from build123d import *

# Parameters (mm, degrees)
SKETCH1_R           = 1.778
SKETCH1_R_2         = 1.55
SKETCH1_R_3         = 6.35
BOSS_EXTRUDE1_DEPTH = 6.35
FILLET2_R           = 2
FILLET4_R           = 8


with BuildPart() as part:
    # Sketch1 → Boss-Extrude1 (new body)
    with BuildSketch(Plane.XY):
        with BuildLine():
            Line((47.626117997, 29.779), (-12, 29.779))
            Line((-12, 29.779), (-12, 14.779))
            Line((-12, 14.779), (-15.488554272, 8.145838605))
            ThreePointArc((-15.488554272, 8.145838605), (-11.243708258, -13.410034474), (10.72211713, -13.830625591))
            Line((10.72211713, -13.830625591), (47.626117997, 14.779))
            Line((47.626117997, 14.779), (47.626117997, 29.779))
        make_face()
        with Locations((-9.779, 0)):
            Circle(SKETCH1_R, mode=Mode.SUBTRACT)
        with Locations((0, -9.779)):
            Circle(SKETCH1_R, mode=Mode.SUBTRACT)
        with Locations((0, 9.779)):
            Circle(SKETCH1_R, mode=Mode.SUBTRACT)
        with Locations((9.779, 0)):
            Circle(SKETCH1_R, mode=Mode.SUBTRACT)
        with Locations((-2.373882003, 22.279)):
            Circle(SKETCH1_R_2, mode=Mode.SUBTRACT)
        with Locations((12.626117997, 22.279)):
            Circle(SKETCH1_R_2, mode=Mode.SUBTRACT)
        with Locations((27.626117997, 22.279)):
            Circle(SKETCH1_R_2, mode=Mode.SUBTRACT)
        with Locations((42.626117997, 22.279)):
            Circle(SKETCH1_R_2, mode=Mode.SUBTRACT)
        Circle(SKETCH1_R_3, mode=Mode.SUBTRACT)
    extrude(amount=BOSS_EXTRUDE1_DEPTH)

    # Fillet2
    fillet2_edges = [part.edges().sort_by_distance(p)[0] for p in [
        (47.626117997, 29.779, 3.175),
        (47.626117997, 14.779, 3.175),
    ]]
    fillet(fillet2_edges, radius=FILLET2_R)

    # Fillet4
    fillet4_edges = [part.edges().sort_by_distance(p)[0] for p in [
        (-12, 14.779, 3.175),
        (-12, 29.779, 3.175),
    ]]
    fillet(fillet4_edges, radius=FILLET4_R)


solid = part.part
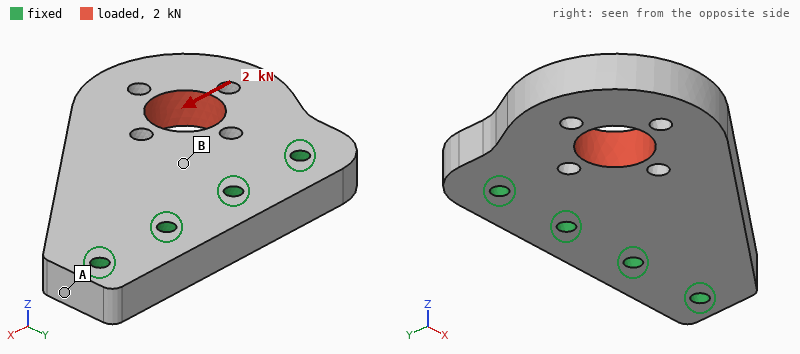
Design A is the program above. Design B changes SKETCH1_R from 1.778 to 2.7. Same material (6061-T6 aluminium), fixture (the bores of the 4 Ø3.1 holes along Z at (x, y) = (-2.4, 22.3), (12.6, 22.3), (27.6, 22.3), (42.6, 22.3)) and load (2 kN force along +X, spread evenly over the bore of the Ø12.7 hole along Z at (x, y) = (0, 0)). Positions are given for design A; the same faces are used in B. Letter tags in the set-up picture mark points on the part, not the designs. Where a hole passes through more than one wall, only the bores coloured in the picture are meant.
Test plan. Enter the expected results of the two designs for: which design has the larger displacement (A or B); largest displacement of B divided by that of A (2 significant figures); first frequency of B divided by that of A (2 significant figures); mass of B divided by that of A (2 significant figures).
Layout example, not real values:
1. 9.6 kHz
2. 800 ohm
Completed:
1. B
2. 1.2
3. 1.00
4. 0.97
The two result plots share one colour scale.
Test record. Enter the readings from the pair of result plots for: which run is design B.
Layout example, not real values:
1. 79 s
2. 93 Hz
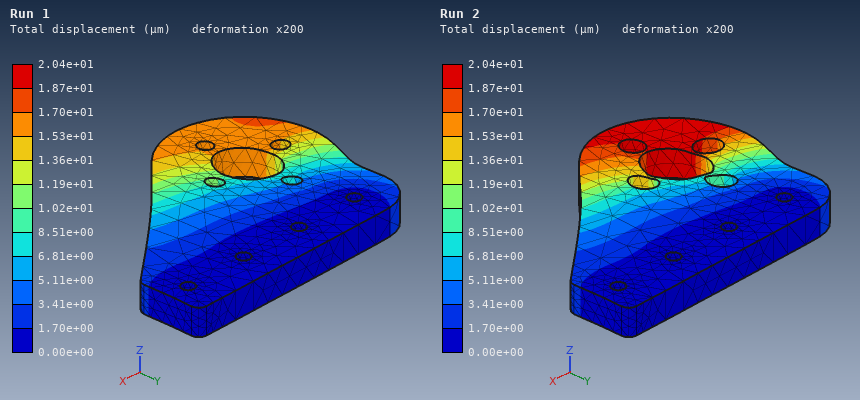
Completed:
1. Run 2
